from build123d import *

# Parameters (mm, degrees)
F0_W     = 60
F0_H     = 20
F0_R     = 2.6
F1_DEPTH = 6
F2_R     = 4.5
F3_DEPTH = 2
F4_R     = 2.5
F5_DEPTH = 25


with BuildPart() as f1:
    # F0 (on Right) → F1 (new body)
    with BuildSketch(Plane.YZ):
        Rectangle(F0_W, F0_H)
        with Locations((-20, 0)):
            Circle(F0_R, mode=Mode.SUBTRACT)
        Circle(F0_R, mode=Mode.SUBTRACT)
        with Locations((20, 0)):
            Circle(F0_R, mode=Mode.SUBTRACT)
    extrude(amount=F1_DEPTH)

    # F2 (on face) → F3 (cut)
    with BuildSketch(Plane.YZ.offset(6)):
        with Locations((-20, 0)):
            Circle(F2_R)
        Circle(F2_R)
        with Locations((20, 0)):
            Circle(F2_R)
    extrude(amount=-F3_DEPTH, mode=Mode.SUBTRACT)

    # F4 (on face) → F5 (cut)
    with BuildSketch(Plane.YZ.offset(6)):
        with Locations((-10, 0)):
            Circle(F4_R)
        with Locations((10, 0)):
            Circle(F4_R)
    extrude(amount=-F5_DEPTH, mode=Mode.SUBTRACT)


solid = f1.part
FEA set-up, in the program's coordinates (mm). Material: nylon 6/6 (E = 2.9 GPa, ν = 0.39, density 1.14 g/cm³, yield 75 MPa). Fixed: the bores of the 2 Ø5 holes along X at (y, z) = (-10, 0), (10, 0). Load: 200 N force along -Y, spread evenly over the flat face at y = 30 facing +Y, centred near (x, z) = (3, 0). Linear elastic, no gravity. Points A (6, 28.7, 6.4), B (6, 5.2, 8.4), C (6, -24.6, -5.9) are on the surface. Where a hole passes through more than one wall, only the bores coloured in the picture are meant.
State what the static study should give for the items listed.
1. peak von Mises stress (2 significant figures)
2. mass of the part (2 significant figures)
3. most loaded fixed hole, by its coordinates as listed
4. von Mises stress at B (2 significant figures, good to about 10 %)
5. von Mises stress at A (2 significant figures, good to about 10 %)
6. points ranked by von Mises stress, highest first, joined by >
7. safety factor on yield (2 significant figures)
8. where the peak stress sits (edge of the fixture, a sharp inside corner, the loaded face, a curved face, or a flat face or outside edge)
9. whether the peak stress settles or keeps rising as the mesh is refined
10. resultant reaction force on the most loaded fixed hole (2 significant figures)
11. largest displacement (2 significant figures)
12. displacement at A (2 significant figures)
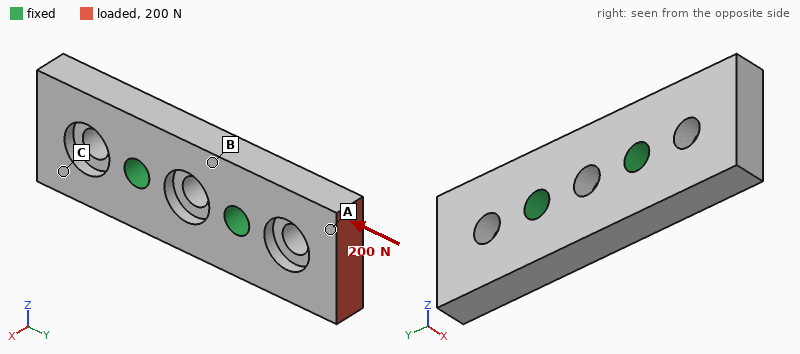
8.2 MPa
7.2 g
(10, 0)
0.96 MPa
1.8 MPa
A > B > C
9.1
a curved face
settles
160 N
26 µm
21 µm
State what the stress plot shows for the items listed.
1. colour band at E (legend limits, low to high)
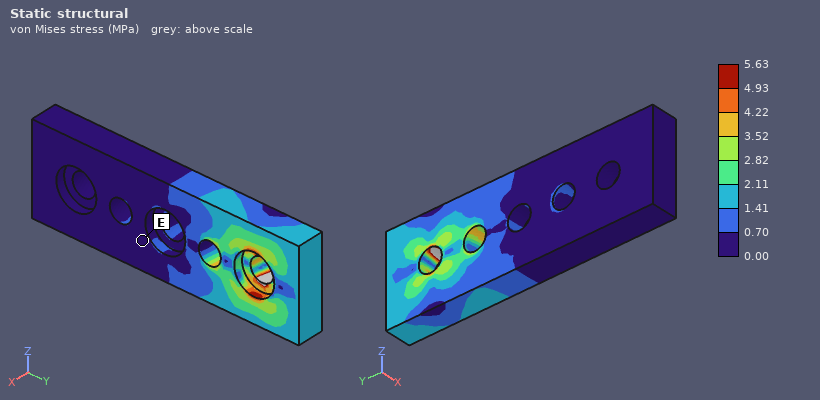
0.00 to 0.70 MPa
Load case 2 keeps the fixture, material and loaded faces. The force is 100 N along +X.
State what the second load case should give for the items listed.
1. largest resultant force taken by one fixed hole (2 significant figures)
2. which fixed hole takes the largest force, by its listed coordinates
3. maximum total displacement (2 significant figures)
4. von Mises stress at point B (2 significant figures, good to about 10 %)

120 N
(10, 0)
0.34 mm
3.4 MPa
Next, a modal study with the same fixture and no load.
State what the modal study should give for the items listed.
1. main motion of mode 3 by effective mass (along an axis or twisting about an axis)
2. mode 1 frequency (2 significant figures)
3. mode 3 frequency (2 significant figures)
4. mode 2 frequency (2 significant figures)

twisting about X
3400 Hz
5600 Hz
3500 Hz
